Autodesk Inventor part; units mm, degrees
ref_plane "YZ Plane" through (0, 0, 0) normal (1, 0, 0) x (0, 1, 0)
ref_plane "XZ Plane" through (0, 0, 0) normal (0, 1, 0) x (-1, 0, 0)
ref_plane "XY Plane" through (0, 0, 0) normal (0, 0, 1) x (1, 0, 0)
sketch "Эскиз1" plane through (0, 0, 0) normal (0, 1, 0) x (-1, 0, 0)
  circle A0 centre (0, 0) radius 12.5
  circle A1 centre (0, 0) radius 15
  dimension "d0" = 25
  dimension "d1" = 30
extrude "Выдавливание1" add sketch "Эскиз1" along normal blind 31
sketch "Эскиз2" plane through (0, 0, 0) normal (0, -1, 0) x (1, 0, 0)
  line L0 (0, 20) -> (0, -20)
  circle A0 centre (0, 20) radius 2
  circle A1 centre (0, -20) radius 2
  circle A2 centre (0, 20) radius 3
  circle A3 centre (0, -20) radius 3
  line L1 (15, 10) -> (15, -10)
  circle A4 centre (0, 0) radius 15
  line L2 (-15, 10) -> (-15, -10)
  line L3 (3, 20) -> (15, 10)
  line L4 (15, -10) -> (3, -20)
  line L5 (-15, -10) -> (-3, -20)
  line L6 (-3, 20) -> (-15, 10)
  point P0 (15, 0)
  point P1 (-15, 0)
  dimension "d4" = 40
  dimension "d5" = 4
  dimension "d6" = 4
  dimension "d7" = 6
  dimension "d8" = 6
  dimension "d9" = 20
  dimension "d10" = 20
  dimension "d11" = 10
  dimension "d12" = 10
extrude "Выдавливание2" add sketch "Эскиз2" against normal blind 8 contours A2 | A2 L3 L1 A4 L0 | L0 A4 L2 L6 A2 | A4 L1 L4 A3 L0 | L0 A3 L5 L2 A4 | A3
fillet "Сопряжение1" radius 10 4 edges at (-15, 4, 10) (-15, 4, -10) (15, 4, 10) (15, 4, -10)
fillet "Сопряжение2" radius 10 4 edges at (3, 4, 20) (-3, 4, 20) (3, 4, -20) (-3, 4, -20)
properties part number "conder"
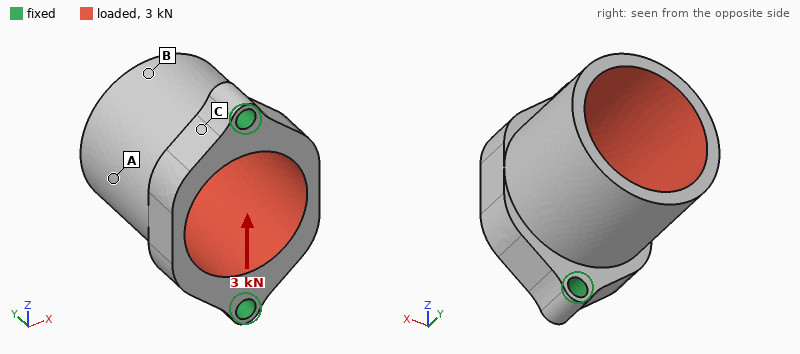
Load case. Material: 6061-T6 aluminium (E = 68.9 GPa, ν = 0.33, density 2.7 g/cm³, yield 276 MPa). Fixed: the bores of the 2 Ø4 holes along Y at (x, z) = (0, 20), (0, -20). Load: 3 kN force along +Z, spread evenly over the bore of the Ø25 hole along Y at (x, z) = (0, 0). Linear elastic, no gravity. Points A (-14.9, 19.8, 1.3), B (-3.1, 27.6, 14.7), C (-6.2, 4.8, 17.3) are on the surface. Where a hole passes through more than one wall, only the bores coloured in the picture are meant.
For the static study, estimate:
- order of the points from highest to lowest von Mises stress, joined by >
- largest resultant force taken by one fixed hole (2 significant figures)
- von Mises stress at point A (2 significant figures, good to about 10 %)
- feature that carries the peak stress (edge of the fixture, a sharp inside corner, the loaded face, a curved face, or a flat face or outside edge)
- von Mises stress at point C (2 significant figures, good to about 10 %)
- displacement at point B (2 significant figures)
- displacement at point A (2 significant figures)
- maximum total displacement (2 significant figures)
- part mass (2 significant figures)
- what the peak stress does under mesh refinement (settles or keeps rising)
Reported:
C > A > B
1.8 kN
20 MPa
edge of the fixture
40 MPa
25 µm
18 µm
27 µm
23 g
keeps rising
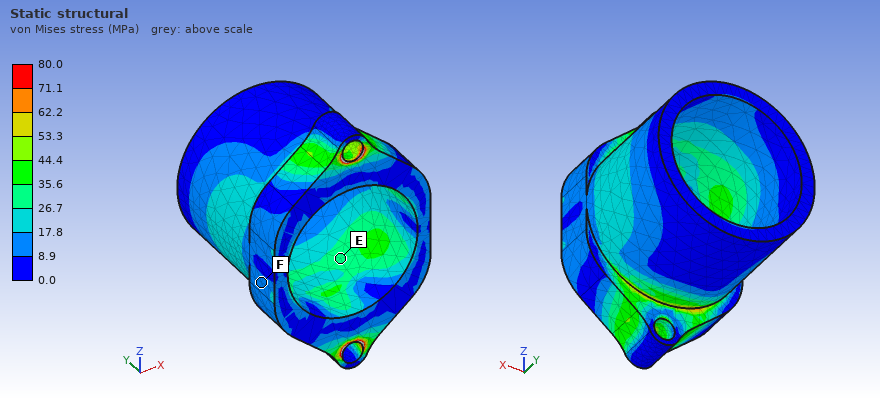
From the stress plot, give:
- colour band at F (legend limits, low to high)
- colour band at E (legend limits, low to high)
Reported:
8.9 to 17.8 MPa
26.7 to 35.6 MPa
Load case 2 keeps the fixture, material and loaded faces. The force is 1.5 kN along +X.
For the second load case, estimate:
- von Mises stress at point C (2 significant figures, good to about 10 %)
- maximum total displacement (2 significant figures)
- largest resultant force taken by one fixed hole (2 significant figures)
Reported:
47 MPa
69 µm
750 N
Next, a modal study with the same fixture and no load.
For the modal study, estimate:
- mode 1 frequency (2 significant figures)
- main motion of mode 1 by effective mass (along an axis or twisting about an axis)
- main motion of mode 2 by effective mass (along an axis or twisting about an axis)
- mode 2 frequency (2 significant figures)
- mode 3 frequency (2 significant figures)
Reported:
5900 Hz
along X
along Y
10 kHz
11 kHz
